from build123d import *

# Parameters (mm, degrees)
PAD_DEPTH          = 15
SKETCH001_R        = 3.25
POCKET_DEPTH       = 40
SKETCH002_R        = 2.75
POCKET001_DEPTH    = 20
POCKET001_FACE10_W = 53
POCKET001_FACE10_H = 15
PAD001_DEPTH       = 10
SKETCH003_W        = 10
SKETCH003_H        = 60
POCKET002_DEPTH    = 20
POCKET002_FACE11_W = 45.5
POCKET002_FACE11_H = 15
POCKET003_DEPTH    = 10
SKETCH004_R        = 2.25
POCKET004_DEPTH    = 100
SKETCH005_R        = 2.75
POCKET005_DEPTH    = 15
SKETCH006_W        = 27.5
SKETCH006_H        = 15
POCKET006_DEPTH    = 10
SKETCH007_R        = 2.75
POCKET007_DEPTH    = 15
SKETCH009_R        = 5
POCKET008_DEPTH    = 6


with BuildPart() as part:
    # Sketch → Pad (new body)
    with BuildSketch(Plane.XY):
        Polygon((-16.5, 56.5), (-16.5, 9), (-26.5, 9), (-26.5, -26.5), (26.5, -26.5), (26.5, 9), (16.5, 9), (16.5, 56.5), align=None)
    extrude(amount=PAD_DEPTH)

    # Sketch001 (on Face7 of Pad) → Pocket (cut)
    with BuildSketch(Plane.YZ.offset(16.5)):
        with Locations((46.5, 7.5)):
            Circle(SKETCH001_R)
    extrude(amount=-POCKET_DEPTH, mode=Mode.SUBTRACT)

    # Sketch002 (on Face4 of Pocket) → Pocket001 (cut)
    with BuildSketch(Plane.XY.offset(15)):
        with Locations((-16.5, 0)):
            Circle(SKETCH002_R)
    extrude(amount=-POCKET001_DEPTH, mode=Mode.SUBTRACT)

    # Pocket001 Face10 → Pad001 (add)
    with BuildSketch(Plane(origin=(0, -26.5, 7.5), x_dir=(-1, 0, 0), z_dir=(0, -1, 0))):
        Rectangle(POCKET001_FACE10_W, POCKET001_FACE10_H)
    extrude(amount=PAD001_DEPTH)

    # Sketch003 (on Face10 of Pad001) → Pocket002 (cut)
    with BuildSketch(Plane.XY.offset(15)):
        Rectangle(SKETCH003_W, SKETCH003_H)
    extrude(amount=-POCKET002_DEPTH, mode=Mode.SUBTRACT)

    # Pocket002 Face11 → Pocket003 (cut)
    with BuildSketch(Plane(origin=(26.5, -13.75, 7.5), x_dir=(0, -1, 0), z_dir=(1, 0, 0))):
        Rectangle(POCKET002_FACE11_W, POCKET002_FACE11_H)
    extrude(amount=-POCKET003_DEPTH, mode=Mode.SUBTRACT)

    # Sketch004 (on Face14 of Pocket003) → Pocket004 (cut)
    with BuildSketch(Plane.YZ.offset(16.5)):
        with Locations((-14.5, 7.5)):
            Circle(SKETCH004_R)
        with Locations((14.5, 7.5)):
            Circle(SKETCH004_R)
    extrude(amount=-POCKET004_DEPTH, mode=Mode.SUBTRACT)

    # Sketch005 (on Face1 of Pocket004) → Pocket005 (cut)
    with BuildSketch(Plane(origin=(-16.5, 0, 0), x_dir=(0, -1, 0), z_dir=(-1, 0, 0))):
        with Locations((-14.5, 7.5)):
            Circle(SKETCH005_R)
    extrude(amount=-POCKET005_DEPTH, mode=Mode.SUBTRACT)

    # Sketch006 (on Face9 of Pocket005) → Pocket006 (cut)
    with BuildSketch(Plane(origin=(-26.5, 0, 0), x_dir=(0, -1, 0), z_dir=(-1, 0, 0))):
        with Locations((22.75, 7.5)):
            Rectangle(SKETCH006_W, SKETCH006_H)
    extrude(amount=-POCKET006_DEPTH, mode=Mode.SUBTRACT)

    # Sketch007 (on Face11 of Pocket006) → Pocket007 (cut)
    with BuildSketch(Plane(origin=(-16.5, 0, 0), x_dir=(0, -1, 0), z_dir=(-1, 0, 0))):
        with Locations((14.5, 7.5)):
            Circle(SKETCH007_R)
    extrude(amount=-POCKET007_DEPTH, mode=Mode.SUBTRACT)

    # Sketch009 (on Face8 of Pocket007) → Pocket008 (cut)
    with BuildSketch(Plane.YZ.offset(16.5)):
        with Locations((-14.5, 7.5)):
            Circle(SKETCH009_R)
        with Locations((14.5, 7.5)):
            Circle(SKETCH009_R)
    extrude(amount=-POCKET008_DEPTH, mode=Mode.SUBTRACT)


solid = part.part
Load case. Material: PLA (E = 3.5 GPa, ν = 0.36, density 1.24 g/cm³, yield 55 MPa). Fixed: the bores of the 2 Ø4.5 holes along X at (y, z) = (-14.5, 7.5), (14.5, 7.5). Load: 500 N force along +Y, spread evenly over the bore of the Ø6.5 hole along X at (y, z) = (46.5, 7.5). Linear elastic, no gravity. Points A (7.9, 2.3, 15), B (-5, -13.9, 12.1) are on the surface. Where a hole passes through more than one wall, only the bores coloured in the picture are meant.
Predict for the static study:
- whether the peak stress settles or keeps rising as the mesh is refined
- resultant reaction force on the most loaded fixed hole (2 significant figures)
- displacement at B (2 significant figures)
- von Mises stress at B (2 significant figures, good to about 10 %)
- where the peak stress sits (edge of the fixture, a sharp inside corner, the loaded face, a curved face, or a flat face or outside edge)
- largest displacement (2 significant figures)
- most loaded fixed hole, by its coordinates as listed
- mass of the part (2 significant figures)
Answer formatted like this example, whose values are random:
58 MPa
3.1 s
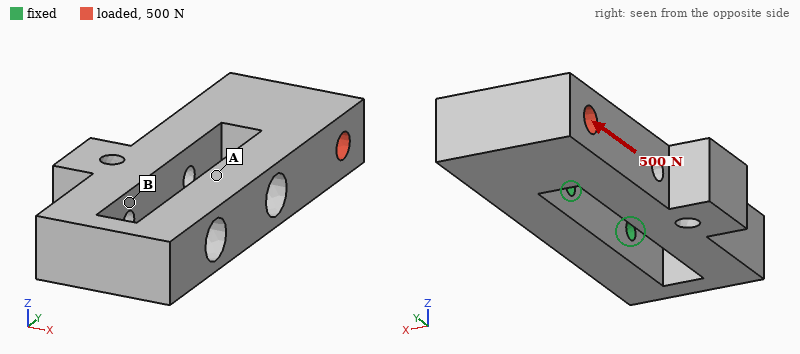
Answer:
keeps rising
360 N
0.13 mm
2.8 MPa
edge of the fixture
0.31 mm
(14.5, 7.5)
45 g
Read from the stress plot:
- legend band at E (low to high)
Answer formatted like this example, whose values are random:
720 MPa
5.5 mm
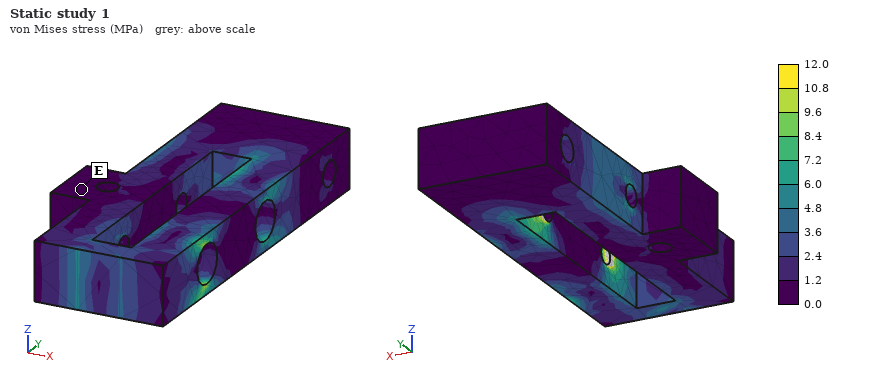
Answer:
0.0 to 1.2 MPa
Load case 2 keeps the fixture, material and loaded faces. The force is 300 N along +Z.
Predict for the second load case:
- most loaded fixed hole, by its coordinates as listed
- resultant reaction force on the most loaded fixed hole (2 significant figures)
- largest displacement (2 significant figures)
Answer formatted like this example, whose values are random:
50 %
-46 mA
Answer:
(14.5, 7.5)
540 N
0.96 mm
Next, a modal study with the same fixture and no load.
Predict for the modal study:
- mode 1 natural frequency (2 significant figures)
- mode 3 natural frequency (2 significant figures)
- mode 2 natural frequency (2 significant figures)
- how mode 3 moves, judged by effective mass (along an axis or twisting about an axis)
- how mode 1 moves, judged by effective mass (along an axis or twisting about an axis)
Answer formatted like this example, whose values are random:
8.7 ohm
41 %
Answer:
720 Hz
1100 Hz
890 Hz
twisting about X
along Z
